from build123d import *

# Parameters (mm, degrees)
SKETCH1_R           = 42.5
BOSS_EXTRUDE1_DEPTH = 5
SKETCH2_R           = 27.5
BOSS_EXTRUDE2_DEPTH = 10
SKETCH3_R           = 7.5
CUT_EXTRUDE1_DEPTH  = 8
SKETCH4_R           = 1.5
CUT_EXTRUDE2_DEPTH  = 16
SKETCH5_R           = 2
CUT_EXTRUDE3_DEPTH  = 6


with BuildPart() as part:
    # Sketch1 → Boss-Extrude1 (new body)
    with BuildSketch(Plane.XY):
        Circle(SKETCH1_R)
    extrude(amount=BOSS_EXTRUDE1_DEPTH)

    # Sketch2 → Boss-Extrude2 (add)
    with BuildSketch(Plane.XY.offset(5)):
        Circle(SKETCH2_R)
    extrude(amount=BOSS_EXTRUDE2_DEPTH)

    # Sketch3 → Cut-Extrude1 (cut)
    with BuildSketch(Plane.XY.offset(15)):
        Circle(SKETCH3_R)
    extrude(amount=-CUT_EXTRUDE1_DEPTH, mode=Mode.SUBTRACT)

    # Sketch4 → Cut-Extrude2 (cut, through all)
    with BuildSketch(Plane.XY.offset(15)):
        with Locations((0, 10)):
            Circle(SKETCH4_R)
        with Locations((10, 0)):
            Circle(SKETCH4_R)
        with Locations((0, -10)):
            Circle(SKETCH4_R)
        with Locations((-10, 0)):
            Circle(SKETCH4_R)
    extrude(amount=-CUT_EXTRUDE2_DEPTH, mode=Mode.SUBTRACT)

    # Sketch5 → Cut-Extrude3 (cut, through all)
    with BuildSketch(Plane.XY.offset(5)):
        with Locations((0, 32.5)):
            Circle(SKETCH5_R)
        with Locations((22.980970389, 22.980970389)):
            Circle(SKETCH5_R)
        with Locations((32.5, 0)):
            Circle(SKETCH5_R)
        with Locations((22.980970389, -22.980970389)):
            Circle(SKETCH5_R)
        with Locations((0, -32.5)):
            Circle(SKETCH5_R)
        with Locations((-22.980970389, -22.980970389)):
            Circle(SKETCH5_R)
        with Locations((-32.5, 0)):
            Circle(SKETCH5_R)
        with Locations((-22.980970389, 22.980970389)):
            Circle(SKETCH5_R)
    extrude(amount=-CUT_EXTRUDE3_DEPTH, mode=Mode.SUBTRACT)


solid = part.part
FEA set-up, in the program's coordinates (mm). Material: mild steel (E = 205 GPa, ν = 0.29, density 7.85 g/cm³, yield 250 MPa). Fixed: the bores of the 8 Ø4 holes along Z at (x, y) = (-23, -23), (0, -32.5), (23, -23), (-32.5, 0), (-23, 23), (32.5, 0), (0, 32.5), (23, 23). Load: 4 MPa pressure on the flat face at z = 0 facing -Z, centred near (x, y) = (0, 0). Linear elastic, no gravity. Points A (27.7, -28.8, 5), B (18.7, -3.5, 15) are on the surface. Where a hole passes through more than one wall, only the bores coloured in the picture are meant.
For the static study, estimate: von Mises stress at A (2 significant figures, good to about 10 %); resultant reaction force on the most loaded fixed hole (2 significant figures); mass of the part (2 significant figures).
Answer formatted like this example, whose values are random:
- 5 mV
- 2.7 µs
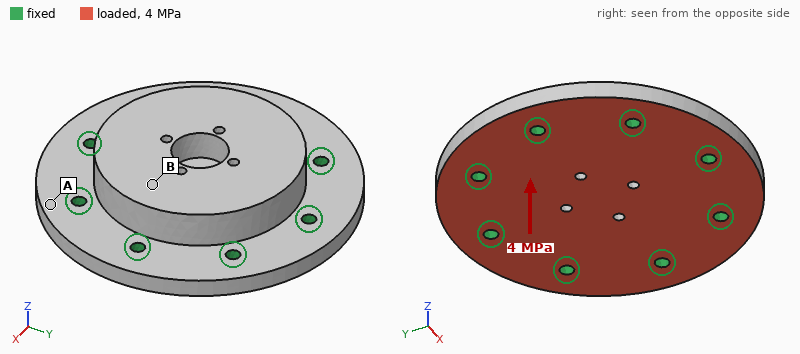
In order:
- 32 MPa
- 2.8 kN
- 390 g
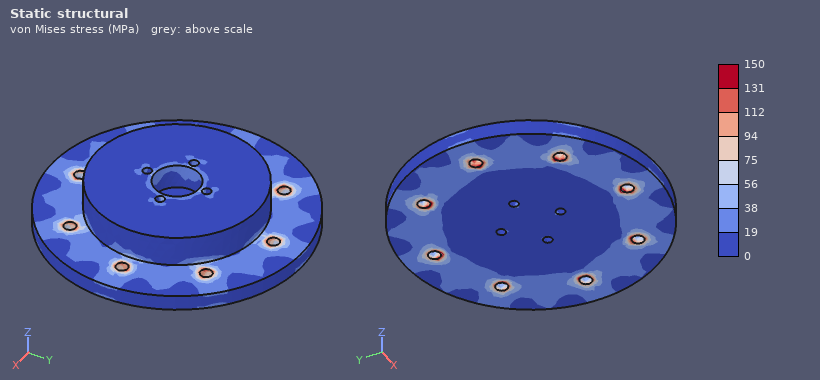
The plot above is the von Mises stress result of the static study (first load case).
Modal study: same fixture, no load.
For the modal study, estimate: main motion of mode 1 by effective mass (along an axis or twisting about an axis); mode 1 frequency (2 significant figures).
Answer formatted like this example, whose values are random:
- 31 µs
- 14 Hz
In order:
- along Z
- 15 kHz
